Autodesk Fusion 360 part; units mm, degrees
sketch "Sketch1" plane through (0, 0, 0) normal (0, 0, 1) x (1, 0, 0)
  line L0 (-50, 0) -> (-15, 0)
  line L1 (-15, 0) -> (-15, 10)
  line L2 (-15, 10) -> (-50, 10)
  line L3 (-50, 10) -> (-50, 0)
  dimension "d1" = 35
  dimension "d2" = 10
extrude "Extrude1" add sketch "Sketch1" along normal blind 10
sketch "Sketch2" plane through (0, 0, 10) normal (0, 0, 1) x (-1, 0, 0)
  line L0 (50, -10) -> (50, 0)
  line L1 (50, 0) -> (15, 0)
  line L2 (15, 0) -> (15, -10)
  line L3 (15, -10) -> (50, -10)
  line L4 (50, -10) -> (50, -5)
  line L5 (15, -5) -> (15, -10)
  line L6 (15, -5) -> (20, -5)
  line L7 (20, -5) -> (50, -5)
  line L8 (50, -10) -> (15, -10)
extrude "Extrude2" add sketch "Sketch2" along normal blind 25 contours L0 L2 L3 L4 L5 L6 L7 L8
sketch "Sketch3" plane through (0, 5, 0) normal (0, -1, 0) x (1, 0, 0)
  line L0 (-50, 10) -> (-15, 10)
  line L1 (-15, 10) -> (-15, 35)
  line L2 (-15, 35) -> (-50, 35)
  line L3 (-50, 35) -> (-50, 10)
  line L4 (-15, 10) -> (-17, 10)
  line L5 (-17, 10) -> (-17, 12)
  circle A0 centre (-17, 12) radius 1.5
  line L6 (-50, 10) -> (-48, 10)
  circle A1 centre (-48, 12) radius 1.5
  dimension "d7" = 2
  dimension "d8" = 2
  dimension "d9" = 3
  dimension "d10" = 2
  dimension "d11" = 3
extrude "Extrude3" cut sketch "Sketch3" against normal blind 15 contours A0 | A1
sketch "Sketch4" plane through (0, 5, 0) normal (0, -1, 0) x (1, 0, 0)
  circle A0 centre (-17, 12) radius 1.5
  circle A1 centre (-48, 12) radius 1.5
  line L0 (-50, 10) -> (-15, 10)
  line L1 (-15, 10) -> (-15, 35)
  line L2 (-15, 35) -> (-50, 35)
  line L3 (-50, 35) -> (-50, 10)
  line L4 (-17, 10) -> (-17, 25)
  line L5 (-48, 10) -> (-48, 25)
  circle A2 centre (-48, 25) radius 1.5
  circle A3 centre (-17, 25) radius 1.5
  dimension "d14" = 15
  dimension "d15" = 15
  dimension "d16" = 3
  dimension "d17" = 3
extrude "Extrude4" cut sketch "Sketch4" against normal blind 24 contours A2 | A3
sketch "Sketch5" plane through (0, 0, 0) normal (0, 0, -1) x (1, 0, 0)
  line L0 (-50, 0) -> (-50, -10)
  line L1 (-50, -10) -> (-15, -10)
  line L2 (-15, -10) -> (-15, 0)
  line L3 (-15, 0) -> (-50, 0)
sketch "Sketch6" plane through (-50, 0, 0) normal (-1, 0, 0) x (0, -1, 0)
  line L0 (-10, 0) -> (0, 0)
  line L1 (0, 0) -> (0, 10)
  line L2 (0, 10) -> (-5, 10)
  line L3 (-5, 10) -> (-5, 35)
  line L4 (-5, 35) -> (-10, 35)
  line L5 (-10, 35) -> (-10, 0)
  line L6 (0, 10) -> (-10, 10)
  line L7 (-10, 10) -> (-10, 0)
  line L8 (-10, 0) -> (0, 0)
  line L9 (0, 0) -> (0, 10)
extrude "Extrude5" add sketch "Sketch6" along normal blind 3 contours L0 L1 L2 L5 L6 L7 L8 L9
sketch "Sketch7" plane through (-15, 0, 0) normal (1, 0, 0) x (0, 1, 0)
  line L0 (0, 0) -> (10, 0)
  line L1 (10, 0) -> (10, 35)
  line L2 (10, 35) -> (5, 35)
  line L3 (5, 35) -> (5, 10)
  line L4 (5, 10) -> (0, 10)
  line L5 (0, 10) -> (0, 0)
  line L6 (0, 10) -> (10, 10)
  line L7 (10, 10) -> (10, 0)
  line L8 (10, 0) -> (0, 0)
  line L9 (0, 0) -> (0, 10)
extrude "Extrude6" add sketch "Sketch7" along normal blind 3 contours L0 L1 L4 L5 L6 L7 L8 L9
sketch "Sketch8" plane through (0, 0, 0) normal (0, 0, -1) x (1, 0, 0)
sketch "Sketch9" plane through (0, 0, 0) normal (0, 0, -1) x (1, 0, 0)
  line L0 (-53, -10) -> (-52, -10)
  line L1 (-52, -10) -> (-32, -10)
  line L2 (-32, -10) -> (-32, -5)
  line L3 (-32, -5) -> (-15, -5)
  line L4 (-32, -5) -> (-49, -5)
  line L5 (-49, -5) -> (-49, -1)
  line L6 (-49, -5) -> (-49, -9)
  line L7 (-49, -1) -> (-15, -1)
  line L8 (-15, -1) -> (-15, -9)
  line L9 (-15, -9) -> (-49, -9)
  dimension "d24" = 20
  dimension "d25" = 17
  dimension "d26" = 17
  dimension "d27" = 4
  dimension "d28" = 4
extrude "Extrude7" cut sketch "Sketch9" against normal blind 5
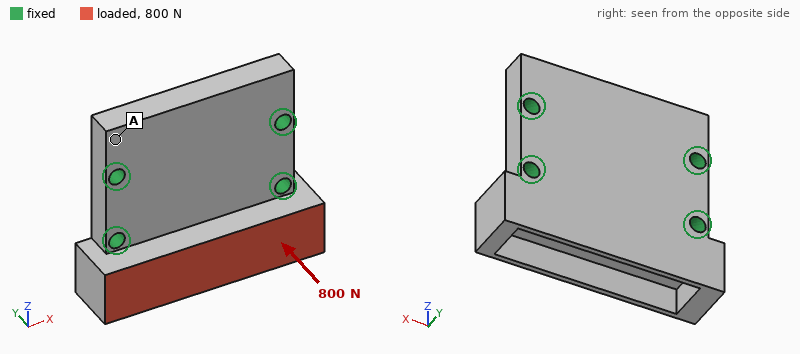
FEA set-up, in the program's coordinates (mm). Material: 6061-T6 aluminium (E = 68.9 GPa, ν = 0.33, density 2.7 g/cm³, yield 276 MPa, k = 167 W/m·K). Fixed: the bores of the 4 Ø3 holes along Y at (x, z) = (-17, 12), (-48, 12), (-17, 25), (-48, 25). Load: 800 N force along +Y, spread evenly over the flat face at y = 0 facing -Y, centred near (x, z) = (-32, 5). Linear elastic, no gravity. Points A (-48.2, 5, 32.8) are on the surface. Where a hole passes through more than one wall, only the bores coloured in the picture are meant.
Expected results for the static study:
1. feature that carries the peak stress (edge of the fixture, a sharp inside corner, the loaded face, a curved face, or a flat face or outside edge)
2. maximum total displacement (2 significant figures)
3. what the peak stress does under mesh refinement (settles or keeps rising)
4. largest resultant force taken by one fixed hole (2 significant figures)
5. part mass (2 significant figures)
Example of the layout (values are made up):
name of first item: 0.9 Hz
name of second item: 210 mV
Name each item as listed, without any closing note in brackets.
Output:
feature that carries the peak stress: edge of the fixture
maximum total displacement: 52 µm
what the peak stress does under mesh refinement: keeps rising
largest resultant force taken by one fixed hole: 460 N
part mass: 19 g
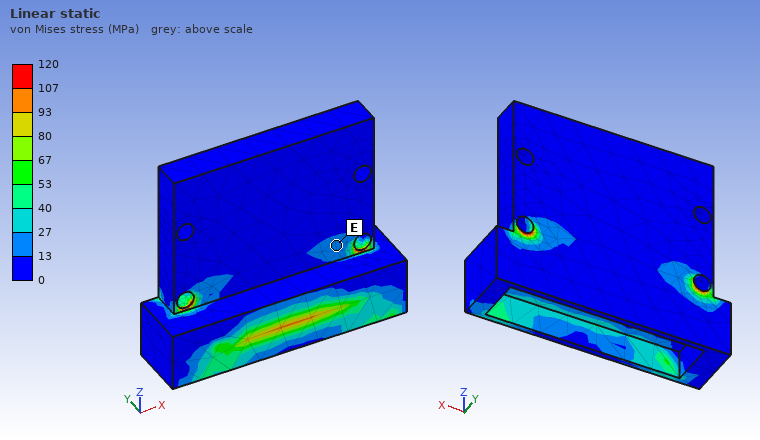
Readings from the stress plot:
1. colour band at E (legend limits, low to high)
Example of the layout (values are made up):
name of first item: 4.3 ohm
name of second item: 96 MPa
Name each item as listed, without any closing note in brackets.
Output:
colour band at E: 13 to 27 MPa
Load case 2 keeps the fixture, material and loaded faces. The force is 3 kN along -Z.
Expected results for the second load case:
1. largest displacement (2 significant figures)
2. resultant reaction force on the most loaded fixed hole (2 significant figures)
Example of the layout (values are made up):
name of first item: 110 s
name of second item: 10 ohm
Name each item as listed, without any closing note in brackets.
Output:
largest displacement: 0.11 mm
resultant reaction force on the most loaded fixed hole: 1.1 kN
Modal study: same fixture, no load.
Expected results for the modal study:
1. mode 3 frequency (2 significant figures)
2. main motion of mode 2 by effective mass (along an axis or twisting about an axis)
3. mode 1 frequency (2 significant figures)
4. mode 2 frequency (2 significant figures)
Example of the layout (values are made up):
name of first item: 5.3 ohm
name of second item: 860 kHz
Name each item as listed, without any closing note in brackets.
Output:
mode 3 frequency: 22 kHz
main motion of mode 2 by effective mass: along Y
mode 1 frequency: 17 kHz
mode 2 frequency: 20 kHz
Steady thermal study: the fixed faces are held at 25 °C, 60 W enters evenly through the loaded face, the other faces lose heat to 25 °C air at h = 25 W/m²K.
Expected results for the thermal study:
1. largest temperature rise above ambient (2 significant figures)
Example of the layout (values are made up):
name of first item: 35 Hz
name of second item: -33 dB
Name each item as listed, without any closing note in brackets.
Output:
largest temperature rise above ambient: 37 K
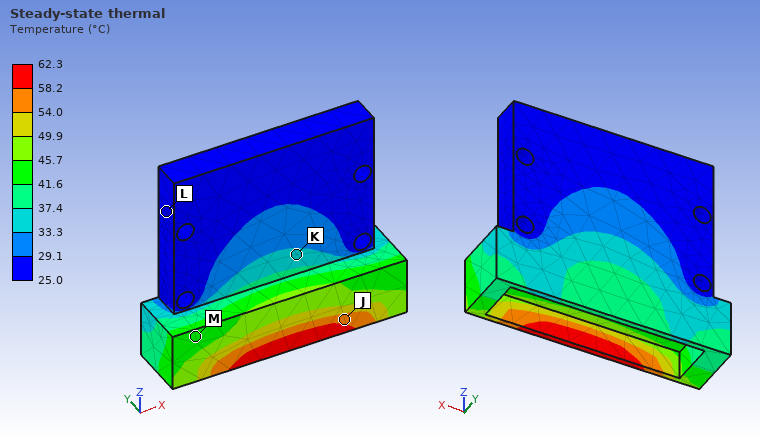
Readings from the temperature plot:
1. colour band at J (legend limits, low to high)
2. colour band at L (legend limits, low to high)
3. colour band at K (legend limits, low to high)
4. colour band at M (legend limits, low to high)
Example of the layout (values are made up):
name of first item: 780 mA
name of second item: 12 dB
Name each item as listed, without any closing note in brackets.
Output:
colour band at J: 54.0 to 58.2 °C
colour band at L: 25.0 to 29.1 °C
colour band at K: 33.3 to 37.4 °C
colour band at M: 41.6 to 45.7 °C
